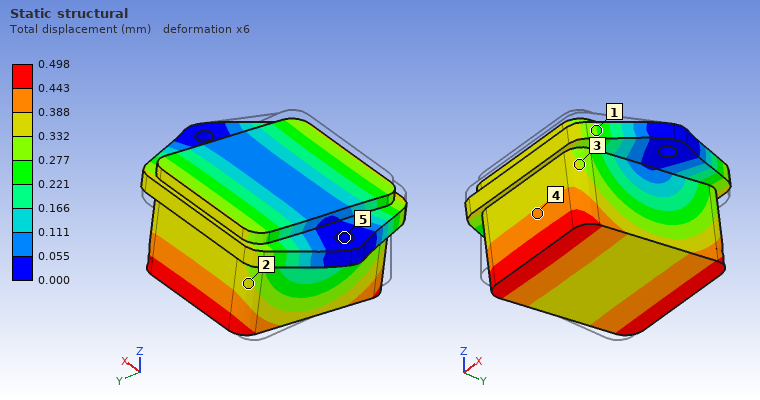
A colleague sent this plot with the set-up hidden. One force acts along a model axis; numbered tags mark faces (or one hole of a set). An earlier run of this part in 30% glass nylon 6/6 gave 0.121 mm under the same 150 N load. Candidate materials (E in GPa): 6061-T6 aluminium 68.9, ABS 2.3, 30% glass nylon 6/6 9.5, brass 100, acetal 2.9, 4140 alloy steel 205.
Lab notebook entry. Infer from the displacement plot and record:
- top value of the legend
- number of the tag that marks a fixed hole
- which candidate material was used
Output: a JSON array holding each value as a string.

["0.498 mm", "5", "ABS"]
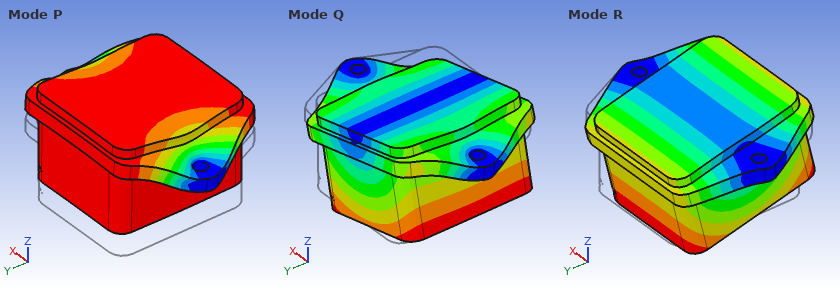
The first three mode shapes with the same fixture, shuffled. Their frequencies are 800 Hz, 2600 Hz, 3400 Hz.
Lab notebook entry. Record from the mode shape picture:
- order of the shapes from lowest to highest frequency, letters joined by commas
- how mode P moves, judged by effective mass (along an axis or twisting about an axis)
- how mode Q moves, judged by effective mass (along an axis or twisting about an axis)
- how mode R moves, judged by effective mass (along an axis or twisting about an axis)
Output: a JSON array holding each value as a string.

["R, P, Q", "along Z", "along X", "along Y"]
